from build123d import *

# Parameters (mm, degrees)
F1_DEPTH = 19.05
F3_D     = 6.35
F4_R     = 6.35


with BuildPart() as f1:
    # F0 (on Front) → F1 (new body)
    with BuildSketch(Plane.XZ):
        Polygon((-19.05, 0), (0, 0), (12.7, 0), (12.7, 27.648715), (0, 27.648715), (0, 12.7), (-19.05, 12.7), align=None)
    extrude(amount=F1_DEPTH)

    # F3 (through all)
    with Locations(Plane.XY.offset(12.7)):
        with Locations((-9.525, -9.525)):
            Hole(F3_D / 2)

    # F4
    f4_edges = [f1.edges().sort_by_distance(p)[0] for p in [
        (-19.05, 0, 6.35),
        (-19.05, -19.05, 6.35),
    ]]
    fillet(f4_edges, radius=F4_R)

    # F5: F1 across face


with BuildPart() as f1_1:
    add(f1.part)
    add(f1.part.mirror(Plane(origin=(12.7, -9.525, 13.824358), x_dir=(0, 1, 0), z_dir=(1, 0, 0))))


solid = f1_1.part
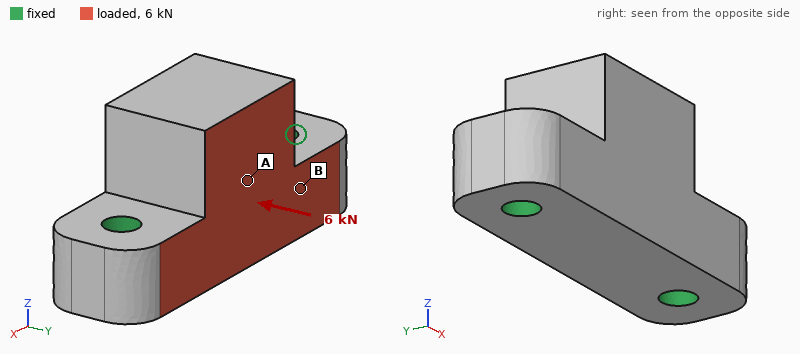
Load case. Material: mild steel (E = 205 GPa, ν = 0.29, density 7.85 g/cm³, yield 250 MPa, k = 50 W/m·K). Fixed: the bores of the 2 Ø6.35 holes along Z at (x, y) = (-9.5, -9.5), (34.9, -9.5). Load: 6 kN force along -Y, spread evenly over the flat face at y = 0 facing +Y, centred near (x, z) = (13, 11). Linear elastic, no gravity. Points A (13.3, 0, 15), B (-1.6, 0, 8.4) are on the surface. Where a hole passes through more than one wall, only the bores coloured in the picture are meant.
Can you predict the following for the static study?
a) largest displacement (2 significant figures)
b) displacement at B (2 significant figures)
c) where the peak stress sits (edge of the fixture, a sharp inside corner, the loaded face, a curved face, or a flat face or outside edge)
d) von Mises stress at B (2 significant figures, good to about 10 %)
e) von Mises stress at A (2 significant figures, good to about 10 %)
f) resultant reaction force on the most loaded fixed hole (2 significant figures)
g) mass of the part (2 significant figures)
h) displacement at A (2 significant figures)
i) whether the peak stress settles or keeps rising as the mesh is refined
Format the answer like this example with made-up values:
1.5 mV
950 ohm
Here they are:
11 µm
3.0 µm
edge of the fixture
37 MPa
13 MPa
3.0 kN
170 g
6.8 µm
keeps rising
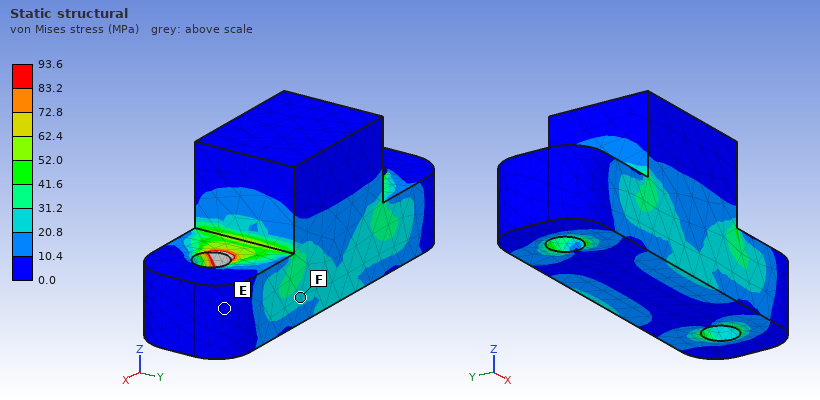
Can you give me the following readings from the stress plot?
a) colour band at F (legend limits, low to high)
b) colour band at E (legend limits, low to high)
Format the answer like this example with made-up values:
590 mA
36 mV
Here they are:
20.8 to 31.2 MPa
0.0 to 10.4 MPa
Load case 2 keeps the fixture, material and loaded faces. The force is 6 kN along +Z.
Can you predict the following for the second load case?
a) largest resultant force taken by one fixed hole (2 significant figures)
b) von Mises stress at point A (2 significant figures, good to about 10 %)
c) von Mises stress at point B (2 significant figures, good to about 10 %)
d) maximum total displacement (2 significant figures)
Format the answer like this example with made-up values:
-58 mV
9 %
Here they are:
3.0 kN
12 MPa
63 MPa
13 µm
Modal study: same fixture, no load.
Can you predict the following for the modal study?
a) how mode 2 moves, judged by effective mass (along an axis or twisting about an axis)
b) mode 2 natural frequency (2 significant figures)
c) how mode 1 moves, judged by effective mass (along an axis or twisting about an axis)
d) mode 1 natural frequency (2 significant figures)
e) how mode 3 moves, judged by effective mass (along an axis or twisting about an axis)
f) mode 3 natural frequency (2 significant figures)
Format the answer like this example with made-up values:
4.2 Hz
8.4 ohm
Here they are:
along Z
20 kHz
along Y
11 kHz
along X
24 kHz
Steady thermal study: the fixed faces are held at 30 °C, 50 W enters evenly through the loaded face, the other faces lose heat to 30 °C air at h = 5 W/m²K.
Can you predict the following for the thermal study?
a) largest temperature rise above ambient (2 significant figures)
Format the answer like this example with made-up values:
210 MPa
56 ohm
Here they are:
34 K
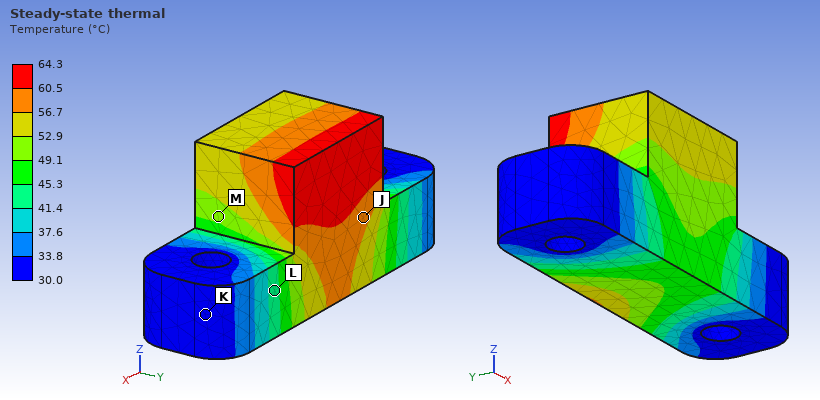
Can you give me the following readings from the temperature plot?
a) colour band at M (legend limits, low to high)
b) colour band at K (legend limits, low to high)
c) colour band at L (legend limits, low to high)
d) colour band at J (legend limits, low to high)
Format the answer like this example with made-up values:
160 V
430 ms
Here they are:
49.1 to 52.9 °C
30.0 to 33.8 °C
41.4 to 45.3 °C
56.7 to 60.5 °C
